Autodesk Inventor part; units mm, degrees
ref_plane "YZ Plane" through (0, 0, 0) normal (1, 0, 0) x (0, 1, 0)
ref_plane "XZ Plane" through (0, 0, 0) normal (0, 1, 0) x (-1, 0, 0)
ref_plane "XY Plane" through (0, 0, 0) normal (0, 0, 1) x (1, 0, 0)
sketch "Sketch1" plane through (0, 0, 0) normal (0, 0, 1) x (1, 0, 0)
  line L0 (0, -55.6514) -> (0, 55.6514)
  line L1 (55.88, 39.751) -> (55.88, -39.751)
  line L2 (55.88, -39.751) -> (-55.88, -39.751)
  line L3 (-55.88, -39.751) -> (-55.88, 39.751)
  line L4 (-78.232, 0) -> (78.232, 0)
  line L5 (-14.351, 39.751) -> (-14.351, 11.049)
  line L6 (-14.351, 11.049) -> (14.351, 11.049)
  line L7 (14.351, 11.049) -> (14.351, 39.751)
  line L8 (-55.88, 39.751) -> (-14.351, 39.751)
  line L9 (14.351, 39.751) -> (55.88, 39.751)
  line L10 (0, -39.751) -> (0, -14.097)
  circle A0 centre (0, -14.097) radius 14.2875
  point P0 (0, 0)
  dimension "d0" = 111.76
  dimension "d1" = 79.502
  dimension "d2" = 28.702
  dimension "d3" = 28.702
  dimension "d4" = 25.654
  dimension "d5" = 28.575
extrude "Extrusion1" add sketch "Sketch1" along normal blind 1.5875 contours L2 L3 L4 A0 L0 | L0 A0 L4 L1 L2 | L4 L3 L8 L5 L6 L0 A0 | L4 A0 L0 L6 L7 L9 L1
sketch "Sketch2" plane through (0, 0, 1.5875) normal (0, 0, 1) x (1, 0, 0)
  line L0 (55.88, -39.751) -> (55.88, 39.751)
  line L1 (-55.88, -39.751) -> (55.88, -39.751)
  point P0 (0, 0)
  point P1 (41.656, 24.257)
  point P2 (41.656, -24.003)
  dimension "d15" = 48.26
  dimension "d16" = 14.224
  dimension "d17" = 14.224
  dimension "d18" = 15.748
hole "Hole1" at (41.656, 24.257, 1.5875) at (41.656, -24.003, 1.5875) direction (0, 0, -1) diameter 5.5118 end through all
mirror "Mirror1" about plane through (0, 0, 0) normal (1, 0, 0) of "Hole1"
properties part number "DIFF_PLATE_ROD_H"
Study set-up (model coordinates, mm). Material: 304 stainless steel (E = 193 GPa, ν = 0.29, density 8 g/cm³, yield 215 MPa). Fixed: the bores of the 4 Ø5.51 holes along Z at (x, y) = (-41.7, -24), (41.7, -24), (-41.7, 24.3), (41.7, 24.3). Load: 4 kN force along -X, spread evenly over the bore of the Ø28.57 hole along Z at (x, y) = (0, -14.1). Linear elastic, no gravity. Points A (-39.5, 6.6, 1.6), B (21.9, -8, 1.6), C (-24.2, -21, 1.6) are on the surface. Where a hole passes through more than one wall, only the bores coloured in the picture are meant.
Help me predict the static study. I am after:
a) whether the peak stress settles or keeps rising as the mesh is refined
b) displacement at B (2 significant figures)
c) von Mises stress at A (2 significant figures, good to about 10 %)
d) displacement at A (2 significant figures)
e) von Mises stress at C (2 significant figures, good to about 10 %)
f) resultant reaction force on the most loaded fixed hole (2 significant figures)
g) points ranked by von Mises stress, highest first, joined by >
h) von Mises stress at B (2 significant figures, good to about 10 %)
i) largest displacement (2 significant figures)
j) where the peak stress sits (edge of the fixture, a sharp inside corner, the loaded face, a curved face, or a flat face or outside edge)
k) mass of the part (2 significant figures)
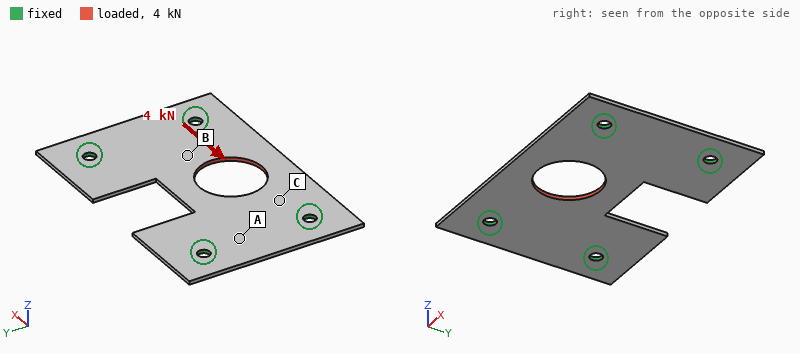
keeps rising
4.4 µm
10 MPa
2.6 µm
36 MPa
1.5 kN
C > B > A
23 MPa
7.1 µm
edge of the fixture
93 g
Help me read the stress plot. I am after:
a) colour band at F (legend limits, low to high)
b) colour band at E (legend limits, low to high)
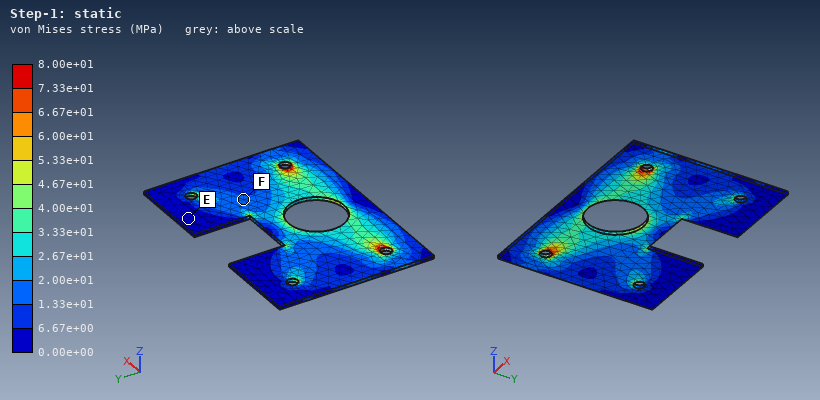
1.33e+01 to 2.00e+01 MPa
0.00e+00 to 6.67e+00 MPa
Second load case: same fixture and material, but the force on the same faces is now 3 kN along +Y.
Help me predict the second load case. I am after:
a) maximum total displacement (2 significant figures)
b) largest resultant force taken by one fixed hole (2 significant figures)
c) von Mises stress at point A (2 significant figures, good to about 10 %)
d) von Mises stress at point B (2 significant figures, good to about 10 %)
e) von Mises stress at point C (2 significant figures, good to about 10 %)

14 µm
990 N
18 MPa
41 MPa
30 MPa
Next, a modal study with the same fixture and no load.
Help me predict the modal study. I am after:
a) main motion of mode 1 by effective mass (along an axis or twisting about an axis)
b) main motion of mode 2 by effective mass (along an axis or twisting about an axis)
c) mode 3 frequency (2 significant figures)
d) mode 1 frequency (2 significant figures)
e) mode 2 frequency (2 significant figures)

along Z
twisting about X
2300 Hz
1300 Hz
1600 Hz
